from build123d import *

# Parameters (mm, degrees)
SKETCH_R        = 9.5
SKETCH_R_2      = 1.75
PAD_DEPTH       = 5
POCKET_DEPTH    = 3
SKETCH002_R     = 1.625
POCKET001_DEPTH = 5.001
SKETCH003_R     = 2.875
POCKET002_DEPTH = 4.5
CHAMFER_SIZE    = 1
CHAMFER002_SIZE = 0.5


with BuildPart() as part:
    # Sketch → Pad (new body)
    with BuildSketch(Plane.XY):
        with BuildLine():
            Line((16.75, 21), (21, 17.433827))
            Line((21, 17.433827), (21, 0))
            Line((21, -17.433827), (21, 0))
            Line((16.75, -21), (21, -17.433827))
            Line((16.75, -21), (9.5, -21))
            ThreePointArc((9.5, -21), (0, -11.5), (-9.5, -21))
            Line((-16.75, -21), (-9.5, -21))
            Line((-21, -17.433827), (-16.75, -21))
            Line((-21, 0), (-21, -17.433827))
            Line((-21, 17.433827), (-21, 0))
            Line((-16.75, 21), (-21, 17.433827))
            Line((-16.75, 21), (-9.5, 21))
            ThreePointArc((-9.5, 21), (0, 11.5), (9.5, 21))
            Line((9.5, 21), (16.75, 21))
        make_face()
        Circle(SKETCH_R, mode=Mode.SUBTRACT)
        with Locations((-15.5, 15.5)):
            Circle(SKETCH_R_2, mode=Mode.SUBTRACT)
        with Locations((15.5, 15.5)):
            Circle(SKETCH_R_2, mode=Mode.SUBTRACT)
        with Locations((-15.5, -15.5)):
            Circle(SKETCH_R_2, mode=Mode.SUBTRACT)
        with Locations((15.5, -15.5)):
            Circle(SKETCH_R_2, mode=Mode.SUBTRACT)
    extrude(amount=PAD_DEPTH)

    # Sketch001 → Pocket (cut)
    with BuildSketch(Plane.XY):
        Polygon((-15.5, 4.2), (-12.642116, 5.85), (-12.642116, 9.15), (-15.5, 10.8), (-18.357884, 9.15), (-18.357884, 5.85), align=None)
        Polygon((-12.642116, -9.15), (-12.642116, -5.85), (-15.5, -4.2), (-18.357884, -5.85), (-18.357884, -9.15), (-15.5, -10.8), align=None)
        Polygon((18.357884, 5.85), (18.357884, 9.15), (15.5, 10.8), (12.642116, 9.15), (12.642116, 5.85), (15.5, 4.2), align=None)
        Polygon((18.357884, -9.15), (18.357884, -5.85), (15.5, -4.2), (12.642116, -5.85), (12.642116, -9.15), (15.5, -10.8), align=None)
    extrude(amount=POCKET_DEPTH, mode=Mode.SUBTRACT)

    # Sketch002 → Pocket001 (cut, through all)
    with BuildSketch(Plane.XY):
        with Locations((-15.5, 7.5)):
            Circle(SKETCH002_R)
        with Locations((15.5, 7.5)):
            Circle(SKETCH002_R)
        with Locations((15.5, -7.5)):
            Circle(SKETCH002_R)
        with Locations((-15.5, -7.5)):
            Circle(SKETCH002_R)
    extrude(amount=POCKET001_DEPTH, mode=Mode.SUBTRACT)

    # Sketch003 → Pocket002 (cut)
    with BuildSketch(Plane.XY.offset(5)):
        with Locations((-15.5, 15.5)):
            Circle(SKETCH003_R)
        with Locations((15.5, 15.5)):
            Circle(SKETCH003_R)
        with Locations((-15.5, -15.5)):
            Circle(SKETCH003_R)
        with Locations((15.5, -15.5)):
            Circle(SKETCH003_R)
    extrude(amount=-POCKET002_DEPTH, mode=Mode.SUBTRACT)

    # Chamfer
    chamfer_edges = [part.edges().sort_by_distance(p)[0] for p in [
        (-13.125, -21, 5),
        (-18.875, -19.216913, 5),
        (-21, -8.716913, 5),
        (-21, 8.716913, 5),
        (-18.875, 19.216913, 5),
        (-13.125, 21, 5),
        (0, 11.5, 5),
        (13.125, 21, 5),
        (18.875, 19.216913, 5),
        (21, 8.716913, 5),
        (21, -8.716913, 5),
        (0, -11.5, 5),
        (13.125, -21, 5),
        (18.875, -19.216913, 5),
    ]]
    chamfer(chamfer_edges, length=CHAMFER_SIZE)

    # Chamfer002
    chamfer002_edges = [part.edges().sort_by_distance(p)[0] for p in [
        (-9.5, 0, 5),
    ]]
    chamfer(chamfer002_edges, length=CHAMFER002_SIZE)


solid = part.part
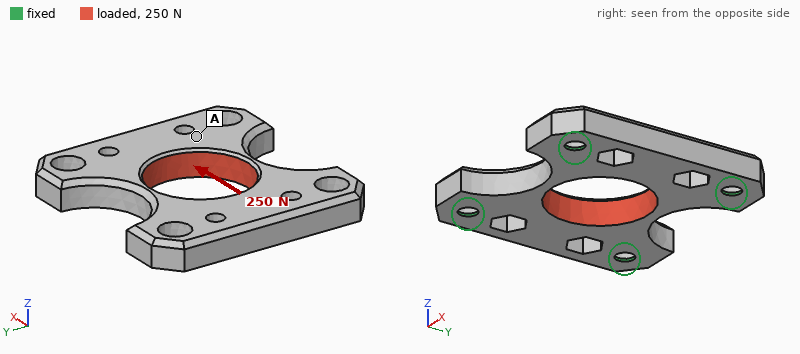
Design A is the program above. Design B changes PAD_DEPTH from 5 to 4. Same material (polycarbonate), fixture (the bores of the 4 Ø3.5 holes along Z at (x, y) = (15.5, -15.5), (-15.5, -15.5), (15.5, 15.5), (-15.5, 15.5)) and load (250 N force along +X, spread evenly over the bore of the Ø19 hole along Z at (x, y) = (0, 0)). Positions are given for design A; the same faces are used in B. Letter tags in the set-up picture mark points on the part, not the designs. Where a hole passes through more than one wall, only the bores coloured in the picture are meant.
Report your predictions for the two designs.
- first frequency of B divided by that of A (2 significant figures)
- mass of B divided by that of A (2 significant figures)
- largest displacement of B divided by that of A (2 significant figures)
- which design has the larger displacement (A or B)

0.90
0.79
1.2
B
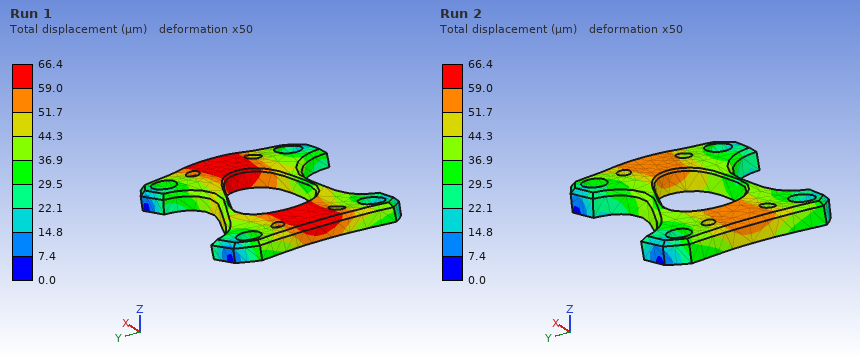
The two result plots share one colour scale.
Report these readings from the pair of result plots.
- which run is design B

Run 1
